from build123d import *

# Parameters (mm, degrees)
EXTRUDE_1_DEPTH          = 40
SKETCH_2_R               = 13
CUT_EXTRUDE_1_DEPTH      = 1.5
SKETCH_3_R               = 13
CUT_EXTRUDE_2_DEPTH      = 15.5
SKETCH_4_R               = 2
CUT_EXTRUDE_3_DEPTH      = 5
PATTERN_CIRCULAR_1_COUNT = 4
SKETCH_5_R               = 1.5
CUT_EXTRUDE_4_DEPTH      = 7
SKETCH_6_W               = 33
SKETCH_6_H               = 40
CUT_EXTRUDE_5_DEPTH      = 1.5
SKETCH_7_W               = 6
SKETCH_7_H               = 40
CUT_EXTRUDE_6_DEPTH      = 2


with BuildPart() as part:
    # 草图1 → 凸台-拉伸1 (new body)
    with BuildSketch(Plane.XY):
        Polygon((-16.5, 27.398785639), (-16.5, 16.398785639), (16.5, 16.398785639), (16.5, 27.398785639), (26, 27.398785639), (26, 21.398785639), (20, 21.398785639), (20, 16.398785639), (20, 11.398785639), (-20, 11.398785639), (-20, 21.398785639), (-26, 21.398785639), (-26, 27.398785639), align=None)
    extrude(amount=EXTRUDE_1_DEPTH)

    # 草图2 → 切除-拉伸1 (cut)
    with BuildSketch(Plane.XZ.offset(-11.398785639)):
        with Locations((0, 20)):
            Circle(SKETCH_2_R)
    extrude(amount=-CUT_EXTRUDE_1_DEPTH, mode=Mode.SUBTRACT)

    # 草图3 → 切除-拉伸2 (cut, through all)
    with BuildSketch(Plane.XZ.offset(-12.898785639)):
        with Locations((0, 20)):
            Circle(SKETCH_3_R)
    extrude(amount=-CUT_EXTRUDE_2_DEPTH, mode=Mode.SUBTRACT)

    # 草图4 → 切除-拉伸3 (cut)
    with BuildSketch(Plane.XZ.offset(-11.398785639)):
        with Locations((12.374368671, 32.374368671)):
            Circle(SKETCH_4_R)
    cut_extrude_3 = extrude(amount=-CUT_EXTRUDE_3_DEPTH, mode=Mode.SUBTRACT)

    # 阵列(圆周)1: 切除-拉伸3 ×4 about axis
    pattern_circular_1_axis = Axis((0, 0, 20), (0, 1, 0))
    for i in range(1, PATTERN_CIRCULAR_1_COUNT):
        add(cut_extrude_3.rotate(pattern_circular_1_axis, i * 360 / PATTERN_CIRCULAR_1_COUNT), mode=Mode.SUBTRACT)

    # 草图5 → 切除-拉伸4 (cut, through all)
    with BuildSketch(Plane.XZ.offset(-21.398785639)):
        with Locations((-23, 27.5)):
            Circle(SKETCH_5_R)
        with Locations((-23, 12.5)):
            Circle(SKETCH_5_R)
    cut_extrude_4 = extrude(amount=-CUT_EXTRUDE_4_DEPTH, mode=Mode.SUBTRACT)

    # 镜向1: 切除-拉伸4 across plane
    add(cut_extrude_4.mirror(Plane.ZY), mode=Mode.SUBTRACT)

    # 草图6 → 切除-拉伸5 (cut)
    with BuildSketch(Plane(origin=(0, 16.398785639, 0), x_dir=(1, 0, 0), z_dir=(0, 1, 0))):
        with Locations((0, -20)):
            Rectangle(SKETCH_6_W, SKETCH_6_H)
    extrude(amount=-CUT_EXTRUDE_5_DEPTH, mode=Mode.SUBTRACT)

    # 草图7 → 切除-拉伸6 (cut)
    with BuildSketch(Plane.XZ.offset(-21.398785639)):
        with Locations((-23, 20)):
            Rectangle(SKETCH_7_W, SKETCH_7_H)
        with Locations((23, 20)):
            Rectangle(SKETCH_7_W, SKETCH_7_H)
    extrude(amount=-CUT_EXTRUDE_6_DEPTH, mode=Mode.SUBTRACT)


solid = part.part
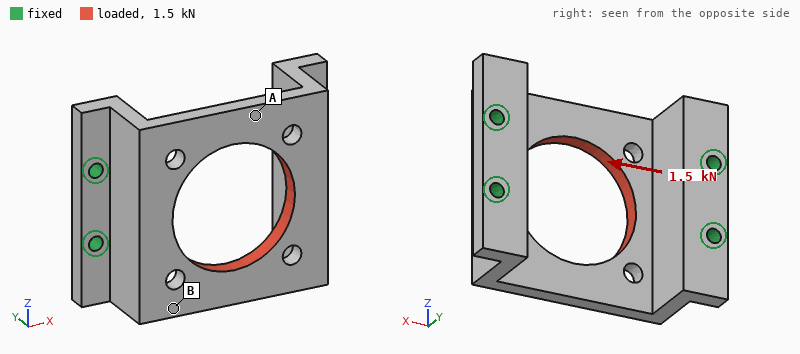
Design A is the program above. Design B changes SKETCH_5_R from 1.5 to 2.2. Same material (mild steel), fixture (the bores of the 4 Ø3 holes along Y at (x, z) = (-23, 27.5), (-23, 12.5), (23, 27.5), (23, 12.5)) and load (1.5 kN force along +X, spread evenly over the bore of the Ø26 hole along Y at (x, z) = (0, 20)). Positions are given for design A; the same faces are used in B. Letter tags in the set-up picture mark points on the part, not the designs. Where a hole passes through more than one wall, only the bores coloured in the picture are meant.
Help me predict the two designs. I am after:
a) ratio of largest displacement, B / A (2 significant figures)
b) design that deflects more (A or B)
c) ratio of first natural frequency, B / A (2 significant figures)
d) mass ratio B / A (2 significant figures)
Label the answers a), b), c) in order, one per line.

a) 0.91
b) A
c) 1.1
d) 0.99
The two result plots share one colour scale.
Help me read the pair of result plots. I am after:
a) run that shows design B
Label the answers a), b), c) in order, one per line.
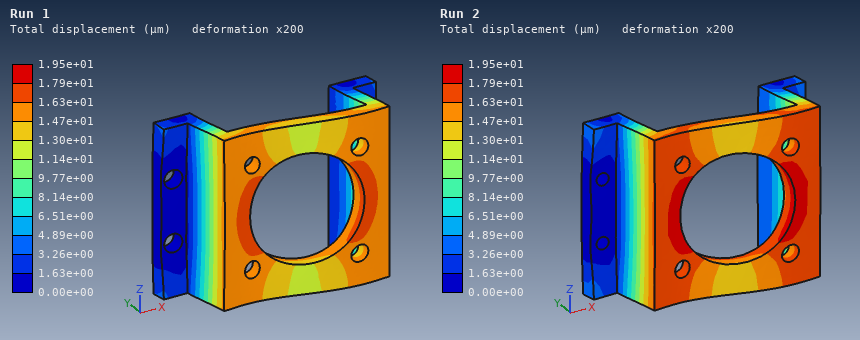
a) Run 1
